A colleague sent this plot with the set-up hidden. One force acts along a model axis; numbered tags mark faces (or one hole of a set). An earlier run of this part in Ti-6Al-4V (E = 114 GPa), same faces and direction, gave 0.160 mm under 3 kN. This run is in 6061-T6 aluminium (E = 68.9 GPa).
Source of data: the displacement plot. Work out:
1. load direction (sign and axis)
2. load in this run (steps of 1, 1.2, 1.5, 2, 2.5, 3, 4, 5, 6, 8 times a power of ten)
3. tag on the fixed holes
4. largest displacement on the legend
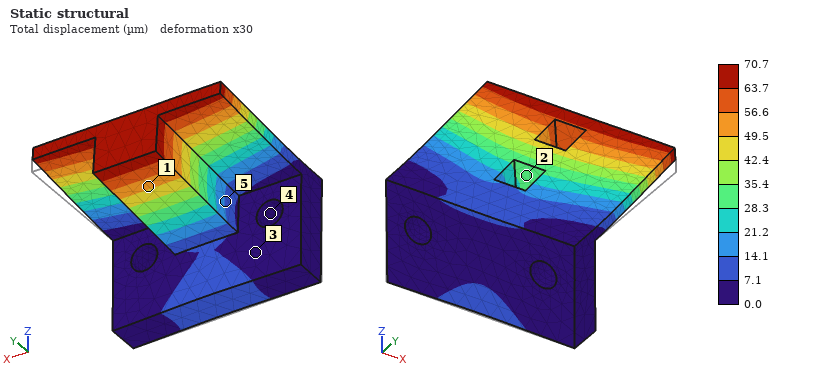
+Z
800 N
4
70.7 µm
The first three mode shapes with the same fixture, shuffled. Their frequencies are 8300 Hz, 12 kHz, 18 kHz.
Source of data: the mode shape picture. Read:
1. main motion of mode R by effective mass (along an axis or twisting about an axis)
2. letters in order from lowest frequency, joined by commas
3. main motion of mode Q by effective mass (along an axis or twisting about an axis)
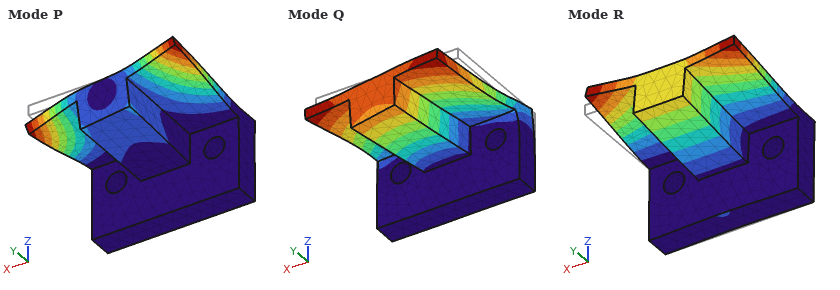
along Z
R, P, Q
along X
